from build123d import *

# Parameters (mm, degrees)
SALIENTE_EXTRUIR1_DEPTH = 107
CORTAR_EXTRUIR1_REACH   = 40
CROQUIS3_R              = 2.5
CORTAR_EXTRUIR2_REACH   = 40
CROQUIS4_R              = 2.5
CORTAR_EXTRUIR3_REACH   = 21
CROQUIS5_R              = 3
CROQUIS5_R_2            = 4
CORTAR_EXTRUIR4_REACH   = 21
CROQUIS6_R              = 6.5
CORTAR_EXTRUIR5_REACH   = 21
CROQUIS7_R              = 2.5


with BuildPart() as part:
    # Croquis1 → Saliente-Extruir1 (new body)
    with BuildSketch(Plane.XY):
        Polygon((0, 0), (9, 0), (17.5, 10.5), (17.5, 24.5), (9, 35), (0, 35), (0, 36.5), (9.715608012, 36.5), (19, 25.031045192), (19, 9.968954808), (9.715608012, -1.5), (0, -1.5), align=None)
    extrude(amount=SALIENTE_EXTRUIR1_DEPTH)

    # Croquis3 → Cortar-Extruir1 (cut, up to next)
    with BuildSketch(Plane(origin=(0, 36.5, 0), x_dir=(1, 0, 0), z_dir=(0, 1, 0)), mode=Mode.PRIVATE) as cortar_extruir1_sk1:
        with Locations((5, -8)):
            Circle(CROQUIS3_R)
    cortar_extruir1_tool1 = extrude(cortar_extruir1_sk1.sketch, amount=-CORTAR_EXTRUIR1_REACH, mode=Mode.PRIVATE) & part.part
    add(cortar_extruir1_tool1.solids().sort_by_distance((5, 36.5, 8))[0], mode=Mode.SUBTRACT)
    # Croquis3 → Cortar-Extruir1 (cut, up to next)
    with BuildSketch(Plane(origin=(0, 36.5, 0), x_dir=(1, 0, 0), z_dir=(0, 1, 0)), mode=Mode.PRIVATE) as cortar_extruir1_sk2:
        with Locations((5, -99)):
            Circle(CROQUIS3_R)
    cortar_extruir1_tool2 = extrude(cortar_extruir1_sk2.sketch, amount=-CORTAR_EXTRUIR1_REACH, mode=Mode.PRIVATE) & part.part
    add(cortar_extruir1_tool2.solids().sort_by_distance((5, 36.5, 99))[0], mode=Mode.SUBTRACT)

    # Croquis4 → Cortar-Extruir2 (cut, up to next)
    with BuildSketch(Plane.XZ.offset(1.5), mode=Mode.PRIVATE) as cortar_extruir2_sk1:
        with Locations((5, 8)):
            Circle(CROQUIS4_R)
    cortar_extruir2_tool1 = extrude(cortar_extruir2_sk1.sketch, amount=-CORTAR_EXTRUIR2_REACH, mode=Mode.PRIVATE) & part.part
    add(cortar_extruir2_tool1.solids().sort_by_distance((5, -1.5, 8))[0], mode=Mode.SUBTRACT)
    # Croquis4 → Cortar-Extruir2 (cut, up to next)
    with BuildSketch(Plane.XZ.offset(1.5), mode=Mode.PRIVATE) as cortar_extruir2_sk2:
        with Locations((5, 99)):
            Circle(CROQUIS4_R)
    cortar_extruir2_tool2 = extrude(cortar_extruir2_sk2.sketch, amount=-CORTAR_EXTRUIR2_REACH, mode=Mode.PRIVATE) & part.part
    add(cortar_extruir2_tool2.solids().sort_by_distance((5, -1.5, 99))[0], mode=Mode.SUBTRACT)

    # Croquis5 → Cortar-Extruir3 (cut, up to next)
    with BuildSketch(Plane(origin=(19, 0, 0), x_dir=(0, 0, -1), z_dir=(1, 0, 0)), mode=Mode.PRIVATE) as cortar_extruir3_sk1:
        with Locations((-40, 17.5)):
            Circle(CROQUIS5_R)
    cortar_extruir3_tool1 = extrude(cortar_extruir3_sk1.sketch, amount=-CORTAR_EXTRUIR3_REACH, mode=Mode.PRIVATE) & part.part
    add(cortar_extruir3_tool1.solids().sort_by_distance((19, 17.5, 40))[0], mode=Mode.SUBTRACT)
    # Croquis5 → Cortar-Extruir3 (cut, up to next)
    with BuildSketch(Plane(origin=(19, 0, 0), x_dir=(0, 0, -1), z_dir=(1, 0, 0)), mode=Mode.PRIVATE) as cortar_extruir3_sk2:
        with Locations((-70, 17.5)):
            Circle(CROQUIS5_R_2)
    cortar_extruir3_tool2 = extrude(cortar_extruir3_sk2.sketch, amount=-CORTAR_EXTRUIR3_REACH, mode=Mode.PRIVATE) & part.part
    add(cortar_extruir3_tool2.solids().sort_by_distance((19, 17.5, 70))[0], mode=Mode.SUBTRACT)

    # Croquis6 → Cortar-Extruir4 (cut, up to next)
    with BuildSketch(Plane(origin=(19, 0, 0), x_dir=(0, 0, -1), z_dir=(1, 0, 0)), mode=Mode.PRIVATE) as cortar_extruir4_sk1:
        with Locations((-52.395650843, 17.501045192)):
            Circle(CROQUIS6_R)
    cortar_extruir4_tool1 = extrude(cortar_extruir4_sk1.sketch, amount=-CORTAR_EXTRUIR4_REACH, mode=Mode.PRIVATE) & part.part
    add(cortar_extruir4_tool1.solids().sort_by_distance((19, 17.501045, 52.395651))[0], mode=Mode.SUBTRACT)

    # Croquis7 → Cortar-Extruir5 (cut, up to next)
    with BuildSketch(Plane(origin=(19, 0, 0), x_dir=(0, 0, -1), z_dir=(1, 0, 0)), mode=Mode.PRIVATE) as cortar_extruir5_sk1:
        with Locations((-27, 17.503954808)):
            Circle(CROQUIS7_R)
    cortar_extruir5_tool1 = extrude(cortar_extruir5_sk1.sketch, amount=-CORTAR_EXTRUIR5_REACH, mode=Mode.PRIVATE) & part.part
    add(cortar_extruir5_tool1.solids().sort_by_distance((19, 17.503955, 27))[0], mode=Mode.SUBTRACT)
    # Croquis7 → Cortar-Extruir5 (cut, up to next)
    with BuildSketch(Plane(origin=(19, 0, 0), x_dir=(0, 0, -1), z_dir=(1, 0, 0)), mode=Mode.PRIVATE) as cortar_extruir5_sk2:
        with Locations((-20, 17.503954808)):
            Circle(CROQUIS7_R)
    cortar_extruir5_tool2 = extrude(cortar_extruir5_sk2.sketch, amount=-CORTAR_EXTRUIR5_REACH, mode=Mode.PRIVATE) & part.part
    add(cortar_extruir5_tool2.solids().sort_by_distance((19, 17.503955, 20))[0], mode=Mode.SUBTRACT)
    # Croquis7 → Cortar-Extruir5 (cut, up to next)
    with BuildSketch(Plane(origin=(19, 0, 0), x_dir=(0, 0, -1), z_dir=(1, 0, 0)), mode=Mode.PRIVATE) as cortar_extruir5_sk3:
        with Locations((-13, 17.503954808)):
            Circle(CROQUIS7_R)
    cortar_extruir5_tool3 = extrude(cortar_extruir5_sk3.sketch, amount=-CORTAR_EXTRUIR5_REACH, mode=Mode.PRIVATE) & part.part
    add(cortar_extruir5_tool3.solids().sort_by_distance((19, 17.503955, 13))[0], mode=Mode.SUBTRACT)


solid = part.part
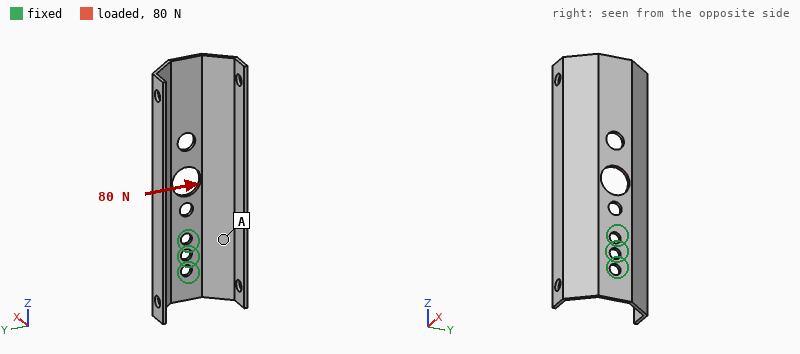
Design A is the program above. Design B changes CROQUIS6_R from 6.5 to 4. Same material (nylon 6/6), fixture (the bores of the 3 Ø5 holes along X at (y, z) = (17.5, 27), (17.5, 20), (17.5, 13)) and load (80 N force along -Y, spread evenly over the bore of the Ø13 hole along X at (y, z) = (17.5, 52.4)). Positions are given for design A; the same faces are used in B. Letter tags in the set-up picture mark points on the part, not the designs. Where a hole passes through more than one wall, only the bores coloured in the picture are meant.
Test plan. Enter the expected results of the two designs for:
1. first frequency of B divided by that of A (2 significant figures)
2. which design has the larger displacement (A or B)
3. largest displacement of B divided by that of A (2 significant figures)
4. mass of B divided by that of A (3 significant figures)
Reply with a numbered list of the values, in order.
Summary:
1. 1.0
2. A
3. 0.90
4. 1.01
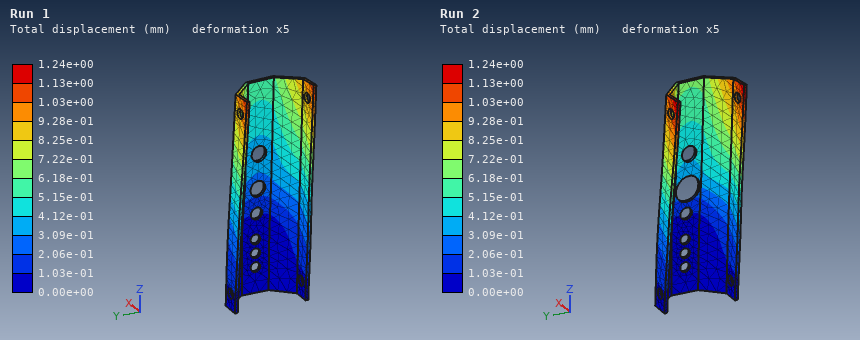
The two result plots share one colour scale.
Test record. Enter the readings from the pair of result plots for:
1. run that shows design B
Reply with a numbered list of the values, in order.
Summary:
1. Run 1
